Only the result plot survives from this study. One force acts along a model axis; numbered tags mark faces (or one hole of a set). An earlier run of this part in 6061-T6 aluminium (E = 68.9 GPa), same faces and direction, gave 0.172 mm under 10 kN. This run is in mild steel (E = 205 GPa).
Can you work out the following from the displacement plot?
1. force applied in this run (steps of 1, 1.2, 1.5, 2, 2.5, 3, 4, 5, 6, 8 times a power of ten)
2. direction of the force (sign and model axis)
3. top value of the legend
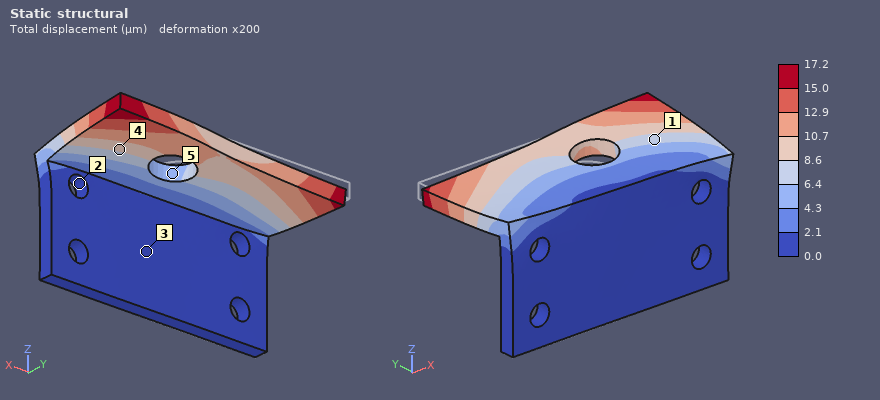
3 kN
+X
17.2 µm
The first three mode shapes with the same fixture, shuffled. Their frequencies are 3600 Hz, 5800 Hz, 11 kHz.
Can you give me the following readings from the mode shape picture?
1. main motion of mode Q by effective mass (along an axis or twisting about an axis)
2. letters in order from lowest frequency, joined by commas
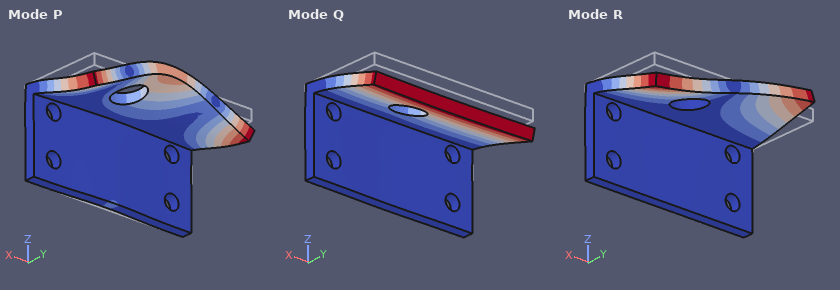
along Z
Q, R, P
